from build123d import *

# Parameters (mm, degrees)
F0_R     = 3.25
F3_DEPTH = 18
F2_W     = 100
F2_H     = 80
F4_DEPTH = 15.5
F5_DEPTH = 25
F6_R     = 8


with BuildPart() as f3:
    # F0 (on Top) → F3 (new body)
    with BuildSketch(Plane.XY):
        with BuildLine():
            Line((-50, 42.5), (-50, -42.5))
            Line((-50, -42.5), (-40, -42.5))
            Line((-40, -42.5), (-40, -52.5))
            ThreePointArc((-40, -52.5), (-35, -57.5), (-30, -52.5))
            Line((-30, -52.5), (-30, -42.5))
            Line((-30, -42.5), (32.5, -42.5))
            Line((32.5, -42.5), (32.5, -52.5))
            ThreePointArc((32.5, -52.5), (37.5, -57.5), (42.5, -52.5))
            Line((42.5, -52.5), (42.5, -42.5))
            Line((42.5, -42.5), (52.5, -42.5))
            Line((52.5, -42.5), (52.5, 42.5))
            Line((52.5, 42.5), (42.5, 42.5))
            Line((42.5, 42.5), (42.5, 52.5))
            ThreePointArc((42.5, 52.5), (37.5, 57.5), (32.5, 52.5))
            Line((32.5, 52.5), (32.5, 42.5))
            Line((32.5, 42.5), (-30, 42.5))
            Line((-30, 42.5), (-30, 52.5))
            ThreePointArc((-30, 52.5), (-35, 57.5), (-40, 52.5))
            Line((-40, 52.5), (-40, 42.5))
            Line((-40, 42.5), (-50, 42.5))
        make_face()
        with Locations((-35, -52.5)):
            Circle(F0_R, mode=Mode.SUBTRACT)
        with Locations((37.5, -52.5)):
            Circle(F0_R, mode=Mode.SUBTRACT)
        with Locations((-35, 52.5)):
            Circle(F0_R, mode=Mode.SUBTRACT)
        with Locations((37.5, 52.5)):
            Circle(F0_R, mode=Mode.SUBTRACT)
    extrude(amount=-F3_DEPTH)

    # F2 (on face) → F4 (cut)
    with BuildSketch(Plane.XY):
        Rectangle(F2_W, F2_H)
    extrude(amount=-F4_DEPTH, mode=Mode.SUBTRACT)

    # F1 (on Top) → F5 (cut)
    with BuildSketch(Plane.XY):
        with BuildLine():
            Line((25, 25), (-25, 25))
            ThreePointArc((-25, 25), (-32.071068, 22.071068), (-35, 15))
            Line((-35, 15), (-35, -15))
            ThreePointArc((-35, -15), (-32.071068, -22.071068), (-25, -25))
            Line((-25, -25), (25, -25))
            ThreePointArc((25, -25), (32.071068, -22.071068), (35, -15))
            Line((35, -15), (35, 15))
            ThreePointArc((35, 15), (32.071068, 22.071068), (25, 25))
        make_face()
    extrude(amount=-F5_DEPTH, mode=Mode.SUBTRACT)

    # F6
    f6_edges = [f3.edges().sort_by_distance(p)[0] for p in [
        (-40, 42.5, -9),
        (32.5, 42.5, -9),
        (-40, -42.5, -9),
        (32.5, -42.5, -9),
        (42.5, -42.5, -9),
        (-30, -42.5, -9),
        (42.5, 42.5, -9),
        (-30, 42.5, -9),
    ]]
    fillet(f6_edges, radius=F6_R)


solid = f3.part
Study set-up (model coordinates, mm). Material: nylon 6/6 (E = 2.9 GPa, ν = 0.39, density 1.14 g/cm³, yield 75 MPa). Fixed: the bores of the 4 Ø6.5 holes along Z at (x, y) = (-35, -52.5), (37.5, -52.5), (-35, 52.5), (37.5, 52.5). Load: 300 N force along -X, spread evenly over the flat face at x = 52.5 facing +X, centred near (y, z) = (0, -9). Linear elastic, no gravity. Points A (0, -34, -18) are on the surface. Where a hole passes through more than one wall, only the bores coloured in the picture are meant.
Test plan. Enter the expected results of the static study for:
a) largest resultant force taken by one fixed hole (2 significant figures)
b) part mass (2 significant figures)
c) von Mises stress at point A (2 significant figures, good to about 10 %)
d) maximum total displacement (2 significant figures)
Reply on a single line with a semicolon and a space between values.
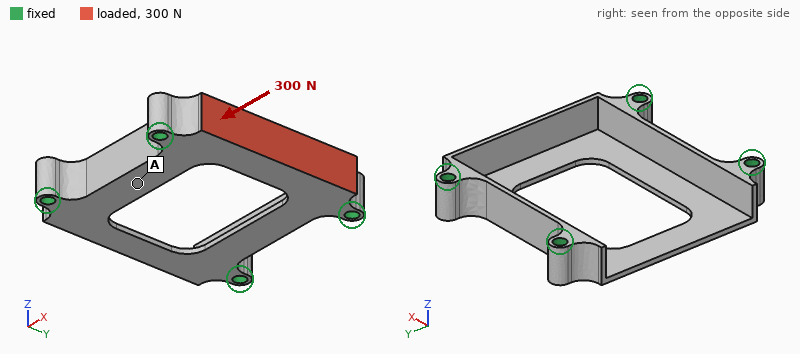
140 N; 39 g; 2.3 MPa; 1.5 mm
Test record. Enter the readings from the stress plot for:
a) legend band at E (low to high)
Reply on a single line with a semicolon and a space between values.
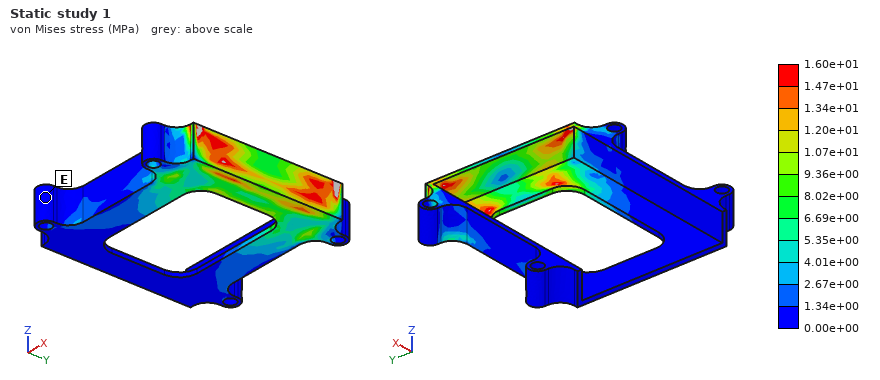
0.00e+00 to 1.34e+00 MPa
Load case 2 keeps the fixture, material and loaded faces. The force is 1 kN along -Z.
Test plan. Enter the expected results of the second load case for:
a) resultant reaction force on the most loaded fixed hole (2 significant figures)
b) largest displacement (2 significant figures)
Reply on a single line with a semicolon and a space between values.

510 N; 1.8 mm
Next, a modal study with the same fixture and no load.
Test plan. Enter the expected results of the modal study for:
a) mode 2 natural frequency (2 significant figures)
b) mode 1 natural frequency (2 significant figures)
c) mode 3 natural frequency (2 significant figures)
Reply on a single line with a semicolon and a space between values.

1200 Hz; 710 Hz; 1600 Hz
